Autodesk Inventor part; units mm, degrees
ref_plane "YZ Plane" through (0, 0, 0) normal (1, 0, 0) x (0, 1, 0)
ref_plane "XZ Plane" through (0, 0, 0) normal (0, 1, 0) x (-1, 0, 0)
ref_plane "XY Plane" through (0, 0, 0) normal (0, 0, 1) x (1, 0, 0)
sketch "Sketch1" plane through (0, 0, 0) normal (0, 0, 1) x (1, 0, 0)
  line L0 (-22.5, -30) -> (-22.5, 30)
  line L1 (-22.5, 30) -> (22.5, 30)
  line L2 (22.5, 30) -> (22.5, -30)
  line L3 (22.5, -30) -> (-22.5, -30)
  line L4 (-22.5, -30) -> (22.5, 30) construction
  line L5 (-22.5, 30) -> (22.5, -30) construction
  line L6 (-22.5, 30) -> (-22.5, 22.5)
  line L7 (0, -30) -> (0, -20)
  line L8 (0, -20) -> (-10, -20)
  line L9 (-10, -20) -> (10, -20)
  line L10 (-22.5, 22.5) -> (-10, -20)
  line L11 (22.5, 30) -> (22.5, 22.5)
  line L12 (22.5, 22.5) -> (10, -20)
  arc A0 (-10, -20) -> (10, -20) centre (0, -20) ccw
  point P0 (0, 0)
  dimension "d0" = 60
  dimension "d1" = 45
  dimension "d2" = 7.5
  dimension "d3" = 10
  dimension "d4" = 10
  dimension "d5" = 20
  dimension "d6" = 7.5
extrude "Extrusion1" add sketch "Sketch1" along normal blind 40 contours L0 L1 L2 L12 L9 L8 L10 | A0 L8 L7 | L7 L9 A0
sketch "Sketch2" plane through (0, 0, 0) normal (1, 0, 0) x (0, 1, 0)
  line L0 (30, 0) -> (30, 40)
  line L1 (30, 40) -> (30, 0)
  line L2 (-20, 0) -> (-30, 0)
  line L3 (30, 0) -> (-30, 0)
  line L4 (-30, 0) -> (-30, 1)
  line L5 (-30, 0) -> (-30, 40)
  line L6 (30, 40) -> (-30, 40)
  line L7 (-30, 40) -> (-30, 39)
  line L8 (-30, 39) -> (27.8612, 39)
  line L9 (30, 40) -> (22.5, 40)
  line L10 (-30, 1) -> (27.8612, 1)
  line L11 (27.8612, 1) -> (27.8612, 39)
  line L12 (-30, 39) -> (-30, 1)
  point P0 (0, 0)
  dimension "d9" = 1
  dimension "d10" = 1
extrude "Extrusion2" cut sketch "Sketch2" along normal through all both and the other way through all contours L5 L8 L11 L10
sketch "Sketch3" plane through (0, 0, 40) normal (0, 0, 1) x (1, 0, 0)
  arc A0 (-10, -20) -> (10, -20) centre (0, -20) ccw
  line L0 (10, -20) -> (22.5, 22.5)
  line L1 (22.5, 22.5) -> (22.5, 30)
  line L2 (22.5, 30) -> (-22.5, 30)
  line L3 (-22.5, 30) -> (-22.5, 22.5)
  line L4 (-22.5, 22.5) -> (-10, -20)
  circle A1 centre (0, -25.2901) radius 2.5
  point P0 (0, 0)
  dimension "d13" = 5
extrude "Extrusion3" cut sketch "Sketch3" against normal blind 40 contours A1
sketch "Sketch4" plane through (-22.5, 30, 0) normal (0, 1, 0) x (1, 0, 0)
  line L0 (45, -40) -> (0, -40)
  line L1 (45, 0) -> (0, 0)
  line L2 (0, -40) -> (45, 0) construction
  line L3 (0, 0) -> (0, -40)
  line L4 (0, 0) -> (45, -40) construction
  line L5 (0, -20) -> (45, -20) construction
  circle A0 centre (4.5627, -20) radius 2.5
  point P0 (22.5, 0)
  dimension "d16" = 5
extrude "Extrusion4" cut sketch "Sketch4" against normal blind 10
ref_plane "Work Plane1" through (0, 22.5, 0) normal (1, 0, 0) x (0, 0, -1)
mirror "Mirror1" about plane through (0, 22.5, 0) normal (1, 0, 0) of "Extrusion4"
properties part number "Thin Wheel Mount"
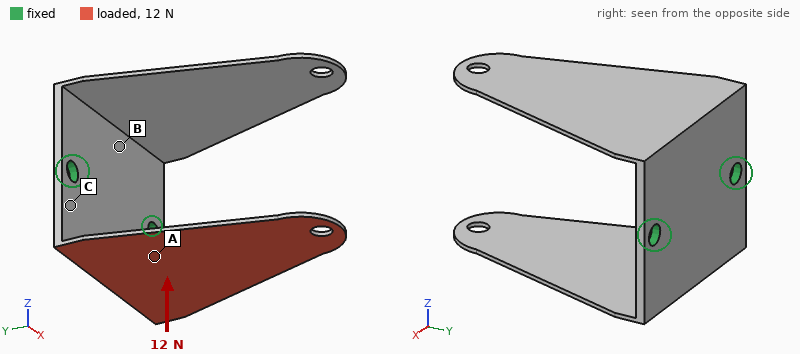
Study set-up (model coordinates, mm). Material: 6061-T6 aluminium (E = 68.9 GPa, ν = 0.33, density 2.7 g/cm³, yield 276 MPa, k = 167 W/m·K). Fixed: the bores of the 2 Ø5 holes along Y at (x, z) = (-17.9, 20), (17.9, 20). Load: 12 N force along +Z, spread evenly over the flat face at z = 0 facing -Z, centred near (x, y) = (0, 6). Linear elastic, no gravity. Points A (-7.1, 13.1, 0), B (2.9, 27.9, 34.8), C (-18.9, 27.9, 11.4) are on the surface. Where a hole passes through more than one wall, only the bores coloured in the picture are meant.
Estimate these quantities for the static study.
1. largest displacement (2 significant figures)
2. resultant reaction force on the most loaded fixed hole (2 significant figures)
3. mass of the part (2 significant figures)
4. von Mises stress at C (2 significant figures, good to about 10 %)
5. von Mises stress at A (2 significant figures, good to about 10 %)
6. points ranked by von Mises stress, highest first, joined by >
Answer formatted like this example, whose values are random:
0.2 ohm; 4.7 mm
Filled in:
0.95 mm; 6.3 N; 20 g; 8.5 MPa; 18 MPa; A > C > B
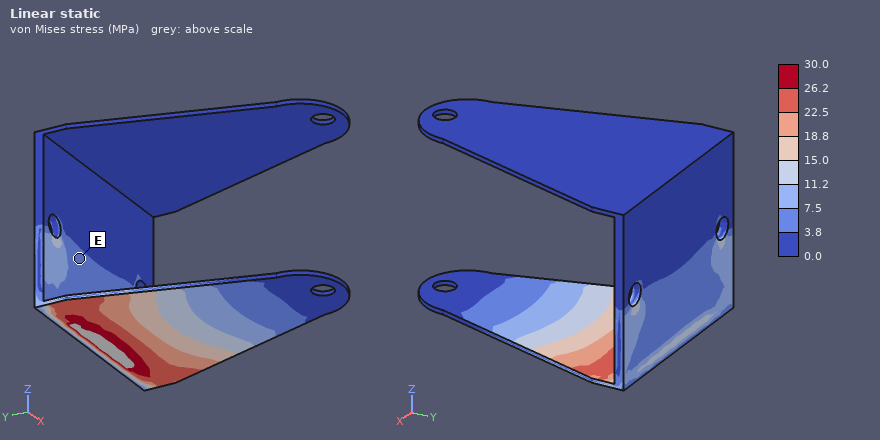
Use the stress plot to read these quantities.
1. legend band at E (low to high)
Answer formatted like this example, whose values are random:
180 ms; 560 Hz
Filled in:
3.8 to 7.5 MPa
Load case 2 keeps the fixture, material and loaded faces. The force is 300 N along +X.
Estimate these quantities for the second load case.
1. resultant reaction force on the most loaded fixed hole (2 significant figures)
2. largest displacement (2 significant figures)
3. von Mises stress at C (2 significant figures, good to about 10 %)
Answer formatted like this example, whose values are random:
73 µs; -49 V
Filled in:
290 N; 0.82 mm; 110 MPa
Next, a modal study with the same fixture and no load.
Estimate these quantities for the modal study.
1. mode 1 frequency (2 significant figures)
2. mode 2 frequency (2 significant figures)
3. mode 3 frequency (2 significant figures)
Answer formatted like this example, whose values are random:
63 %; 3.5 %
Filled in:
340 Hz; 340 Hz; 1400 Hz
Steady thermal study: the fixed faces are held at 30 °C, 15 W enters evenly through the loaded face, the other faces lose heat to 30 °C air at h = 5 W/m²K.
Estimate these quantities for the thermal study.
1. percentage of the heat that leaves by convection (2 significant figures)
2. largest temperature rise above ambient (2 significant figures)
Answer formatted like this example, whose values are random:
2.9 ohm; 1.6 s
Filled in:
4.4 %; 74 K
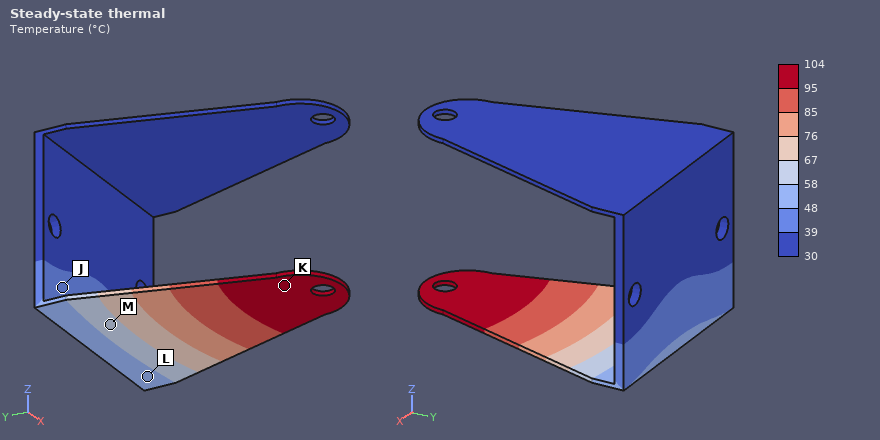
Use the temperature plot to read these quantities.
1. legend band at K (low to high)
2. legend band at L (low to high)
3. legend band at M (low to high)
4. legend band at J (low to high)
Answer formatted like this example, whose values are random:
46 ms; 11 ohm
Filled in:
95 to 104 °C; 48 to 58 °C; 58 to 67 °C; 39 to 48 °C
